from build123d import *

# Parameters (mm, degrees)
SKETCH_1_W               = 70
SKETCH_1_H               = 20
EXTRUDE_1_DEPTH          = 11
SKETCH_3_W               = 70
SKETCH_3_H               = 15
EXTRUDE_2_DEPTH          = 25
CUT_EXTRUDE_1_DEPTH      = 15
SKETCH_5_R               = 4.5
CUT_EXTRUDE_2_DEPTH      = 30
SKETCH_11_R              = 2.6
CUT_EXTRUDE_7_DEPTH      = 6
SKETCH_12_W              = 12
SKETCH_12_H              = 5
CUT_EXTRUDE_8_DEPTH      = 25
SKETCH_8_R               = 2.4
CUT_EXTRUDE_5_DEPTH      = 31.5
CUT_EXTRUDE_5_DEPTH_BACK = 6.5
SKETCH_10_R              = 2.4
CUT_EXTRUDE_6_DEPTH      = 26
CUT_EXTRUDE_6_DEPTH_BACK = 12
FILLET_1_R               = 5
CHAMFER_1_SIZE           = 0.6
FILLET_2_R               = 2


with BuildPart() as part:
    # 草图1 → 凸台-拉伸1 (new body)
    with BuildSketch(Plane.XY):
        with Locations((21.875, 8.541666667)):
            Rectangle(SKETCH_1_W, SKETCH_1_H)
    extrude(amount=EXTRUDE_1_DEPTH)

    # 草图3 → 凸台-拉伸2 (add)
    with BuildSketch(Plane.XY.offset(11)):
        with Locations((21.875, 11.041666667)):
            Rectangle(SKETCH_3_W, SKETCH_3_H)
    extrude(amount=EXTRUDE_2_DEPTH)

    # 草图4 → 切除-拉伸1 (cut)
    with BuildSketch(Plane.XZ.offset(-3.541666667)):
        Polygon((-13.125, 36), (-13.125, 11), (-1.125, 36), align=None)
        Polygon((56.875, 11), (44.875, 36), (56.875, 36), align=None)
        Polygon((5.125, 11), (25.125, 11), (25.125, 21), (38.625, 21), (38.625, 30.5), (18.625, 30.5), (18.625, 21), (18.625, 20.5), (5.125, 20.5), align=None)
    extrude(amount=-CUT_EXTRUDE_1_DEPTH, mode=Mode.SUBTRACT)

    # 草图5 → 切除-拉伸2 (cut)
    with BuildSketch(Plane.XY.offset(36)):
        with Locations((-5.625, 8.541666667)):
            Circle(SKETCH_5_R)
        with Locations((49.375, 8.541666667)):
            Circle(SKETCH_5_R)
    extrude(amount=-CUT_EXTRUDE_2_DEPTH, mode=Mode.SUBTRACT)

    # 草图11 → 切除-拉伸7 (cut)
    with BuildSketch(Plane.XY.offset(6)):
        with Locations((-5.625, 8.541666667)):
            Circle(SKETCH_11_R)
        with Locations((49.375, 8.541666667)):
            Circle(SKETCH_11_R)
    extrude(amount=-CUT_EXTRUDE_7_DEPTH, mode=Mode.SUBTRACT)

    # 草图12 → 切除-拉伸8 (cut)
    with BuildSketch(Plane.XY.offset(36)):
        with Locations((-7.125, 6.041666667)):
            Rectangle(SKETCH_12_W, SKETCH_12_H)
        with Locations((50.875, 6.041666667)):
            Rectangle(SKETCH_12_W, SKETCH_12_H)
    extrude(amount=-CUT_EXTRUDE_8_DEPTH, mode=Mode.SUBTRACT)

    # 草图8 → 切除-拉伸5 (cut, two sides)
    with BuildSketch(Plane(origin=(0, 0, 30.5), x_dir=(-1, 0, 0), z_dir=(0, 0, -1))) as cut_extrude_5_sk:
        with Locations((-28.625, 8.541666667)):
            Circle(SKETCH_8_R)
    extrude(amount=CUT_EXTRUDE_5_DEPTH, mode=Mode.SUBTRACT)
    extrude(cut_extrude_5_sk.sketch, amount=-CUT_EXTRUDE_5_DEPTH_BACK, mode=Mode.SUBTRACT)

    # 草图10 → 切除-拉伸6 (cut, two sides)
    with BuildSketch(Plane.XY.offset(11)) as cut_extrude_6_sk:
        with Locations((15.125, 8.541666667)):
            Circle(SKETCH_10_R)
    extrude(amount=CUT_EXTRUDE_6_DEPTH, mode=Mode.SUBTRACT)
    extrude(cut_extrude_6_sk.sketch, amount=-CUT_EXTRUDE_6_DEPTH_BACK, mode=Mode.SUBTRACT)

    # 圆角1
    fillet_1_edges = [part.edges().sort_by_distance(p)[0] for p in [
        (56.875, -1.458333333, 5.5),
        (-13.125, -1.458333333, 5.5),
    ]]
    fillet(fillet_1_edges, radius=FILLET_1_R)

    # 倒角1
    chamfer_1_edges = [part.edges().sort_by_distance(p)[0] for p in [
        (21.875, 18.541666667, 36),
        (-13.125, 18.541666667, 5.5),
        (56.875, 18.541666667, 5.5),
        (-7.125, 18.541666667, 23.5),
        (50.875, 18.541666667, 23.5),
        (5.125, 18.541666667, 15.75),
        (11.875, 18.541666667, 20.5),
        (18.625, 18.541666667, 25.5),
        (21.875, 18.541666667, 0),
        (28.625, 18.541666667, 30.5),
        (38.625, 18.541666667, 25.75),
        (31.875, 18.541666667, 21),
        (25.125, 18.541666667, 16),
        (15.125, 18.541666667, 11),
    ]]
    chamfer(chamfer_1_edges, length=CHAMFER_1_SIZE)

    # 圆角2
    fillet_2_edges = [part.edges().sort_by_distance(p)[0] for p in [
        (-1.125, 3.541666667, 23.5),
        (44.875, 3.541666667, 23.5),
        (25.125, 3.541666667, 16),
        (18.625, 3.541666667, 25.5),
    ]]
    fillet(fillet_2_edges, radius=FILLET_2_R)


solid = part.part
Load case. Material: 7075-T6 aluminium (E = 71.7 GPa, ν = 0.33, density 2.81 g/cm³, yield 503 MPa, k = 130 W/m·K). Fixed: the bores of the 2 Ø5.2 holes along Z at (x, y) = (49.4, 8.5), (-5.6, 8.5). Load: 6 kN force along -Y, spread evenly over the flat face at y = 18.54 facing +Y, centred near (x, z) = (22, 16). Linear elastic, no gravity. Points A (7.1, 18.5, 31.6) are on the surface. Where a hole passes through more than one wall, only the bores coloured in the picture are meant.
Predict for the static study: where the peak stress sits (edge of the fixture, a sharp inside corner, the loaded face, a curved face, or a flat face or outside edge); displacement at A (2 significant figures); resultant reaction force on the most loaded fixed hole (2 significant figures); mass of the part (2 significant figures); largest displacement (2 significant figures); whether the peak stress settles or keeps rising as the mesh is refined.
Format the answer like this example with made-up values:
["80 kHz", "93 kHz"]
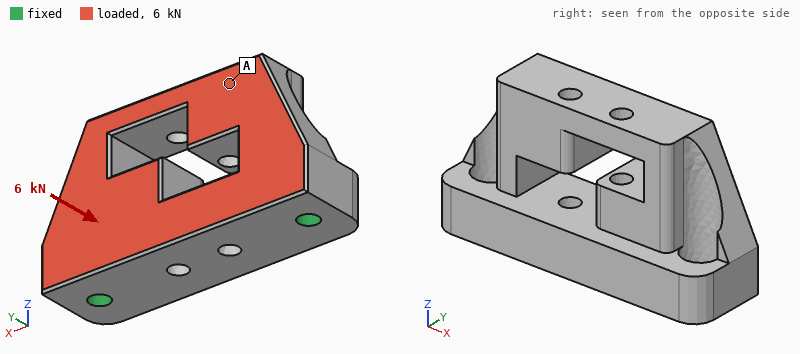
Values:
["edge of the fixture", "0.14 mm", "3.0 kN", "75 g", "0.17 mm", "keeps rising"]
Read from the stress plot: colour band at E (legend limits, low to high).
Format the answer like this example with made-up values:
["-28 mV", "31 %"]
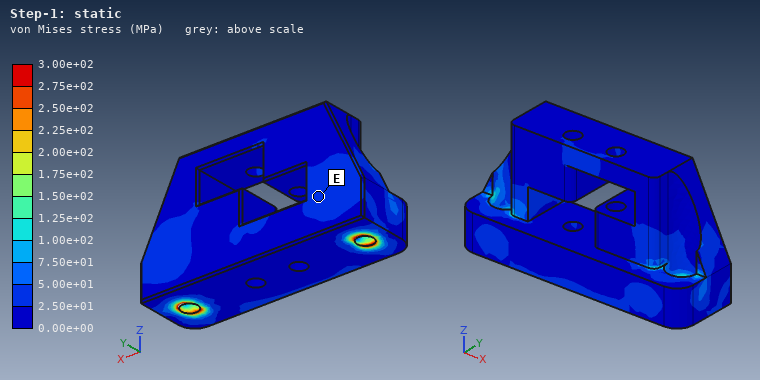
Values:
["2.50e+01 to 5.00e+01 MPa"]
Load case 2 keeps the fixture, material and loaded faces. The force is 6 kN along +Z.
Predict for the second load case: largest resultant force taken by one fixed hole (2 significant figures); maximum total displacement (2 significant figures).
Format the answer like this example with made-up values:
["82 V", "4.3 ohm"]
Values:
["3.1 kN", "0.11 mm"]
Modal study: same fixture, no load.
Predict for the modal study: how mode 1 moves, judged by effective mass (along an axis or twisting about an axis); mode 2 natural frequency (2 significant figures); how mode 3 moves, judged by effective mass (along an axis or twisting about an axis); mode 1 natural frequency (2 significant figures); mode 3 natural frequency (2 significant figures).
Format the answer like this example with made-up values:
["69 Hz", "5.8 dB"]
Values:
["along Y", "9400 Hz", "along X", "4500 Hz", "9900 Hz"]
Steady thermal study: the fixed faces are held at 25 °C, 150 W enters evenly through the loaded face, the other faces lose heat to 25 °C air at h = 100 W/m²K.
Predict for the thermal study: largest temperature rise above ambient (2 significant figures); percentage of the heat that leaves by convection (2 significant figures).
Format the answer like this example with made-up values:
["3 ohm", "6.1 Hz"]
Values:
["51 K", "16 %"]
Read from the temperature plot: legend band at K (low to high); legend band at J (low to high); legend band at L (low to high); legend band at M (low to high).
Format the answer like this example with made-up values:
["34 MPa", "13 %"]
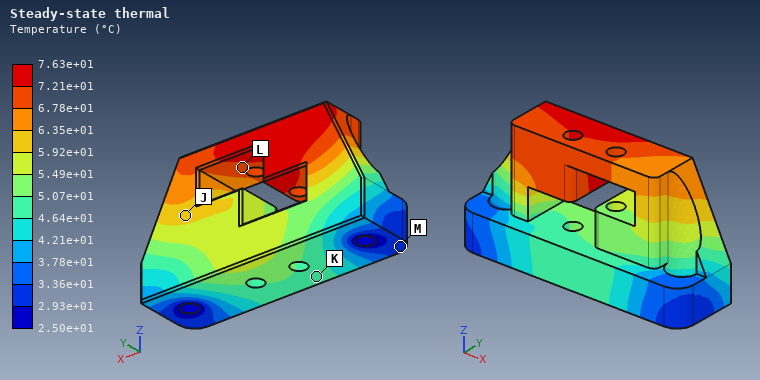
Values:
["4.64e+01 to 5.07e+01 °C", "5.92e+01 to 6.35e+01 °C", "6.78e+01 to 7.21e+01 °C", "2.93e+01 to 3.36e+01 °C"]
